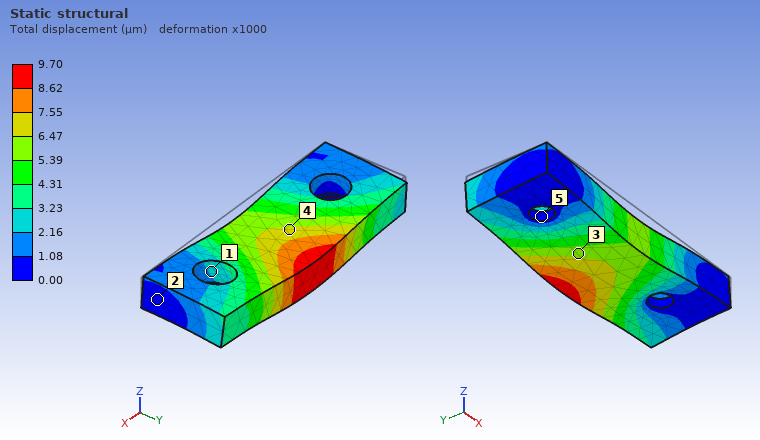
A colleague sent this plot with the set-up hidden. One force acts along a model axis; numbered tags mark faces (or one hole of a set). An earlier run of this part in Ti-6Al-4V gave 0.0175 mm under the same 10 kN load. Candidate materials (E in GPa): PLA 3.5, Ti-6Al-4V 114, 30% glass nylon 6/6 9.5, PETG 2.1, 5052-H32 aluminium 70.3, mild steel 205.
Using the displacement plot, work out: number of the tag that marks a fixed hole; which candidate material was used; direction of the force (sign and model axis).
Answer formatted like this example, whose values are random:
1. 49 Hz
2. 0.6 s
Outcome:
1. 5
2. mild steel
3. -Z
